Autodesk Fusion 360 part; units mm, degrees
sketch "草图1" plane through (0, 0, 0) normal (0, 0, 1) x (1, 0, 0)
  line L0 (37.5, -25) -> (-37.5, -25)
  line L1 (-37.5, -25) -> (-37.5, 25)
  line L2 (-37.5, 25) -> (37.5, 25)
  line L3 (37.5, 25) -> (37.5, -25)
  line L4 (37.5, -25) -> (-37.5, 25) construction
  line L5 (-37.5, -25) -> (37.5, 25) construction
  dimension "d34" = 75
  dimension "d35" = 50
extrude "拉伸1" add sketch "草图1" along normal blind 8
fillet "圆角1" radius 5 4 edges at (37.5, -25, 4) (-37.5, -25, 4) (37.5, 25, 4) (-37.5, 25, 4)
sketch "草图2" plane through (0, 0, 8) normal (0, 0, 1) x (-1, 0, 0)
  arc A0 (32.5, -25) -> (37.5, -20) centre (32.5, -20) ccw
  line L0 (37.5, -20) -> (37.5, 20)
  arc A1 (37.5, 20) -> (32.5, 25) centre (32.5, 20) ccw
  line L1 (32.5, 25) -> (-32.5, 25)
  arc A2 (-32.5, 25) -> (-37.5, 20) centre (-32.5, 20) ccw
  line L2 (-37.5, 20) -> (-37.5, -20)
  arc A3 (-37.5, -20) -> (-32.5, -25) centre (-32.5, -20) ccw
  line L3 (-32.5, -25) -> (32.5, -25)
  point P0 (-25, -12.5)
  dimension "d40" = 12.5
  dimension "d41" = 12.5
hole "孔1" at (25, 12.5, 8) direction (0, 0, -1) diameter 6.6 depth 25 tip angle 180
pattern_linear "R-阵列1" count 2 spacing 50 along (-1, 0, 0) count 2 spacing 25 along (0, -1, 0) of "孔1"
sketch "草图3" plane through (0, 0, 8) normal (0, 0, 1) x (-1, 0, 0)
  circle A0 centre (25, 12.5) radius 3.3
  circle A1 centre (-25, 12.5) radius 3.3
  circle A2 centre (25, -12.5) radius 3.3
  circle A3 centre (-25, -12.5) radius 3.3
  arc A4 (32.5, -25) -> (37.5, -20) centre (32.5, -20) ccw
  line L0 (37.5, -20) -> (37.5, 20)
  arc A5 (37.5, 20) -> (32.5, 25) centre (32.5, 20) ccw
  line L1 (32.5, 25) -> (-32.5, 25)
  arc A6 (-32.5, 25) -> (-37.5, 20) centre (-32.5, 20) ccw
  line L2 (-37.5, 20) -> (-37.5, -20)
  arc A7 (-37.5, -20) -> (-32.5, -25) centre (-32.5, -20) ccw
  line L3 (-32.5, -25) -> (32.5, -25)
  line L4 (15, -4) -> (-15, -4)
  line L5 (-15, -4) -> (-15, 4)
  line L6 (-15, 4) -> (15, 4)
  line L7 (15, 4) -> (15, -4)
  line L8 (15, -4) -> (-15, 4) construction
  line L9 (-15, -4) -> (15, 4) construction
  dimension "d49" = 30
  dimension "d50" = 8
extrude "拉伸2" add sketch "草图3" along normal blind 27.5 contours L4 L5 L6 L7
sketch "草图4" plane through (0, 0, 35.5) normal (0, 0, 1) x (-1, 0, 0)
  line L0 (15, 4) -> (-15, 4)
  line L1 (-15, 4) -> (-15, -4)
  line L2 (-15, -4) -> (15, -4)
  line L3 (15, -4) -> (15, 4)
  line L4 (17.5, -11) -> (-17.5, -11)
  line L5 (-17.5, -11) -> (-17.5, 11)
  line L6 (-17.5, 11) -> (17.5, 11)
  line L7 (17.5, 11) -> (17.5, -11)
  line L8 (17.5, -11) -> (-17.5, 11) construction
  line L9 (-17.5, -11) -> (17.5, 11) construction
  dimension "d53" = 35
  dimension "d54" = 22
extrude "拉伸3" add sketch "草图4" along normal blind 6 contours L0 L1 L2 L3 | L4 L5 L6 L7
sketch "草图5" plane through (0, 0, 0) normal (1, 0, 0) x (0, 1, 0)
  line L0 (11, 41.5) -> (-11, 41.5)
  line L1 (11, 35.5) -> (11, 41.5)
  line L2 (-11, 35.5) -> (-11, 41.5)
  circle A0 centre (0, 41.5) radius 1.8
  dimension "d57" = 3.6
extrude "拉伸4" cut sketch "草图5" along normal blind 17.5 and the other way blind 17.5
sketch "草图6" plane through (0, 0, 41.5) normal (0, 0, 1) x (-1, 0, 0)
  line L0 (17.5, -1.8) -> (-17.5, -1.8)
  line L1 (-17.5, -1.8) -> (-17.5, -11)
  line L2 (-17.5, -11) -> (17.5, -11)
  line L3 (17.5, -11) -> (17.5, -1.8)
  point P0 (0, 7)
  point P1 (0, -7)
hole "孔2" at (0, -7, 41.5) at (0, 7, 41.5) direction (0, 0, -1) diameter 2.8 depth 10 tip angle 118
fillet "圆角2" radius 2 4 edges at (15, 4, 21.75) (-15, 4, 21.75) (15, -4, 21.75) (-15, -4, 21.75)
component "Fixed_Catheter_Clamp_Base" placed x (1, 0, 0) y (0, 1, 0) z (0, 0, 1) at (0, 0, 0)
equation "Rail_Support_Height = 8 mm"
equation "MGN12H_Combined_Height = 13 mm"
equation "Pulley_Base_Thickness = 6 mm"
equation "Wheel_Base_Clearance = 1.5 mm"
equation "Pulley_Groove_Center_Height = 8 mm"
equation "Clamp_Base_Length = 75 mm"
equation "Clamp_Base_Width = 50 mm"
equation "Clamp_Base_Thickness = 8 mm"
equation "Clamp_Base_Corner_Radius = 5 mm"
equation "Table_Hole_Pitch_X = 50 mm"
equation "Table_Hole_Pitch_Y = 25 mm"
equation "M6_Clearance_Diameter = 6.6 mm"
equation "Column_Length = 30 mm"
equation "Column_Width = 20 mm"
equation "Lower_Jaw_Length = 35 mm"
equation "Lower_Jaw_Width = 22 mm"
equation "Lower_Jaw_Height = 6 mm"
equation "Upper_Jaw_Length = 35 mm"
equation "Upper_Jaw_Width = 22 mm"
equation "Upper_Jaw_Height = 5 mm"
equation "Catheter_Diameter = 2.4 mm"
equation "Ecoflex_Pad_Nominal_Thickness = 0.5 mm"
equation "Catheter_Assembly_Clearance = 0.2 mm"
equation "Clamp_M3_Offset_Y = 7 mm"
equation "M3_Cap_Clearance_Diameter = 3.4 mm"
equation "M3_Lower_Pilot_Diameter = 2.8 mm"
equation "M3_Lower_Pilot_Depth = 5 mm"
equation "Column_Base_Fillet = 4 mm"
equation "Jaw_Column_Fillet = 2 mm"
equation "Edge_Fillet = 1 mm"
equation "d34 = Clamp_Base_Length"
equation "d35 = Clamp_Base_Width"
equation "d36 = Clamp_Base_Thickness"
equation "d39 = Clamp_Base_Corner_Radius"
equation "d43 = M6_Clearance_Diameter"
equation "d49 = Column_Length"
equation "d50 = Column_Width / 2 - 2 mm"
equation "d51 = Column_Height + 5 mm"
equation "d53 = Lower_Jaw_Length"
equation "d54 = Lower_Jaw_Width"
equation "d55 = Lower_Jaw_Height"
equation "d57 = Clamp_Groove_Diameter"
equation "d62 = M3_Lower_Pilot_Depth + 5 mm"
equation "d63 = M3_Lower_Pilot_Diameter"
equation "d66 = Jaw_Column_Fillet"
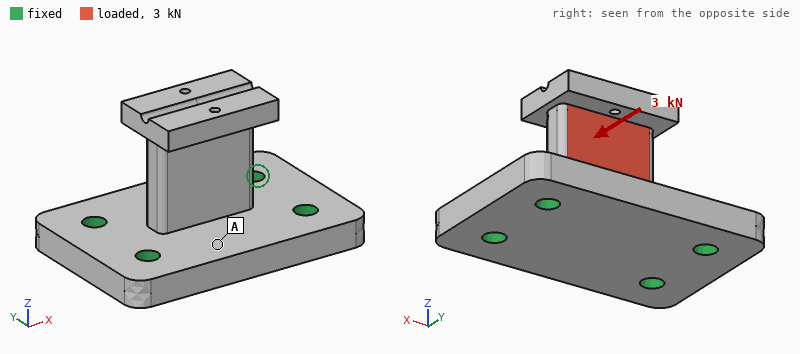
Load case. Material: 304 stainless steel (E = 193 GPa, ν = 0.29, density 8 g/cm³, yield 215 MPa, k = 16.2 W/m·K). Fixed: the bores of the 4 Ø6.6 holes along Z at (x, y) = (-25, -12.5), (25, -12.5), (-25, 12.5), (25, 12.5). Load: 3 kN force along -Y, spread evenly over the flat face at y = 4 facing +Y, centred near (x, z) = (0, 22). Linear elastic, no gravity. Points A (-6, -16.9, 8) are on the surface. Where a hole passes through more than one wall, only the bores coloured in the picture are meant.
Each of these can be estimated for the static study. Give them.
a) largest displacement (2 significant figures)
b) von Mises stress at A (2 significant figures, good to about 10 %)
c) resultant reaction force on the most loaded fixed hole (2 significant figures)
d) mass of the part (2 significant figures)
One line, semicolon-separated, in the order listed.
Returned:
79 µm; 13 MPa; 1.3 kN; 320 g
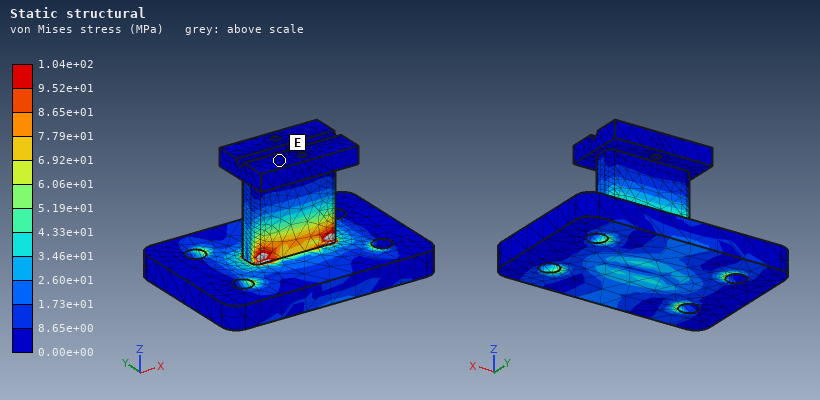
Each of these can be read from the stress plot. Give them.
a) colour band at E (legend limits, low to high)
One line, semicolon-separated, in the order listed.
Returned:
0.00e+00 to 8.65e+00 MPa
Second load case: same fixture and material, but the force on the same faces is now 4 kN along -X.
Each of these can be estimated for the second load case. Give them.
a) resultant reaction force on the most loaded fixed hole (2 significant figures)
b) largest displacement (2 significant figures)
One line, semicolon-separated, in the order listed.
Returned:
1.5 kN; 26 µm
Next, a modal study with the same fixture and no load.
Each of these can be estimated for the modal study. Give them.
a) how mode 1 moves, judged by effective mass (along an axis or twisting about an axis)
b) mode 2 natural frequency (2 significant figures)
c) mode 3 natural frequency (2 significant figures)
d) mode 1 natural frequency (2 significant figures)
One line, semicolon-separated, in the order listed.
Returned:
along Y; 7100 Hz; 7200 Hz; 3000 Hz
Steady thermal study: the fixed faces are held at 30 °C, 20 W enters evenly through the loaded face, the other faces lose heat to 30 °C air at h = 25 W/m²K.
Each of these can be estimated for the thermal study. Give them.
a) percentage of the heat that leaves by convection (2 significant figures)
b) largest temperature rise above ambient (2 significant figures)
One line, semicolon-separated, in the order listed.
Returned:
35 %; 78 K
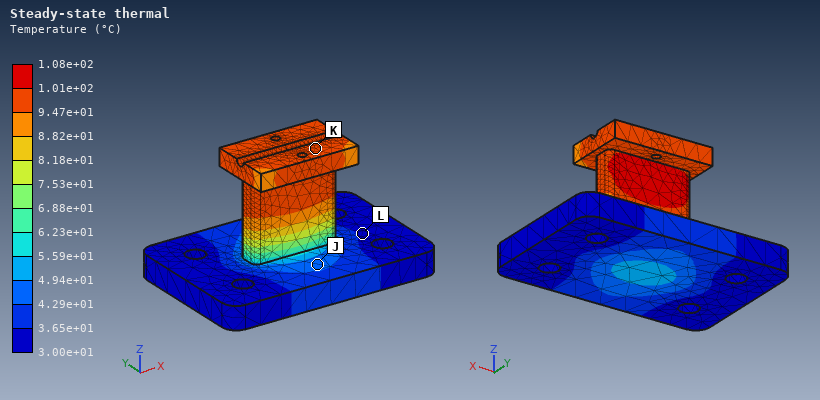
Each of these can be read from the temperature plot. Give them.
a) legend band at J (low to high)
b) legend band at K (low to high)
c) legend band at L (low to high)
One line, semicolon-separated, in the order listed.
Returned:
4.29e+01 to 4.94e+01 °C; 9.47e+01 to 1.01e+02 °C; 3.00e+01 to 3.65e+01 °C
